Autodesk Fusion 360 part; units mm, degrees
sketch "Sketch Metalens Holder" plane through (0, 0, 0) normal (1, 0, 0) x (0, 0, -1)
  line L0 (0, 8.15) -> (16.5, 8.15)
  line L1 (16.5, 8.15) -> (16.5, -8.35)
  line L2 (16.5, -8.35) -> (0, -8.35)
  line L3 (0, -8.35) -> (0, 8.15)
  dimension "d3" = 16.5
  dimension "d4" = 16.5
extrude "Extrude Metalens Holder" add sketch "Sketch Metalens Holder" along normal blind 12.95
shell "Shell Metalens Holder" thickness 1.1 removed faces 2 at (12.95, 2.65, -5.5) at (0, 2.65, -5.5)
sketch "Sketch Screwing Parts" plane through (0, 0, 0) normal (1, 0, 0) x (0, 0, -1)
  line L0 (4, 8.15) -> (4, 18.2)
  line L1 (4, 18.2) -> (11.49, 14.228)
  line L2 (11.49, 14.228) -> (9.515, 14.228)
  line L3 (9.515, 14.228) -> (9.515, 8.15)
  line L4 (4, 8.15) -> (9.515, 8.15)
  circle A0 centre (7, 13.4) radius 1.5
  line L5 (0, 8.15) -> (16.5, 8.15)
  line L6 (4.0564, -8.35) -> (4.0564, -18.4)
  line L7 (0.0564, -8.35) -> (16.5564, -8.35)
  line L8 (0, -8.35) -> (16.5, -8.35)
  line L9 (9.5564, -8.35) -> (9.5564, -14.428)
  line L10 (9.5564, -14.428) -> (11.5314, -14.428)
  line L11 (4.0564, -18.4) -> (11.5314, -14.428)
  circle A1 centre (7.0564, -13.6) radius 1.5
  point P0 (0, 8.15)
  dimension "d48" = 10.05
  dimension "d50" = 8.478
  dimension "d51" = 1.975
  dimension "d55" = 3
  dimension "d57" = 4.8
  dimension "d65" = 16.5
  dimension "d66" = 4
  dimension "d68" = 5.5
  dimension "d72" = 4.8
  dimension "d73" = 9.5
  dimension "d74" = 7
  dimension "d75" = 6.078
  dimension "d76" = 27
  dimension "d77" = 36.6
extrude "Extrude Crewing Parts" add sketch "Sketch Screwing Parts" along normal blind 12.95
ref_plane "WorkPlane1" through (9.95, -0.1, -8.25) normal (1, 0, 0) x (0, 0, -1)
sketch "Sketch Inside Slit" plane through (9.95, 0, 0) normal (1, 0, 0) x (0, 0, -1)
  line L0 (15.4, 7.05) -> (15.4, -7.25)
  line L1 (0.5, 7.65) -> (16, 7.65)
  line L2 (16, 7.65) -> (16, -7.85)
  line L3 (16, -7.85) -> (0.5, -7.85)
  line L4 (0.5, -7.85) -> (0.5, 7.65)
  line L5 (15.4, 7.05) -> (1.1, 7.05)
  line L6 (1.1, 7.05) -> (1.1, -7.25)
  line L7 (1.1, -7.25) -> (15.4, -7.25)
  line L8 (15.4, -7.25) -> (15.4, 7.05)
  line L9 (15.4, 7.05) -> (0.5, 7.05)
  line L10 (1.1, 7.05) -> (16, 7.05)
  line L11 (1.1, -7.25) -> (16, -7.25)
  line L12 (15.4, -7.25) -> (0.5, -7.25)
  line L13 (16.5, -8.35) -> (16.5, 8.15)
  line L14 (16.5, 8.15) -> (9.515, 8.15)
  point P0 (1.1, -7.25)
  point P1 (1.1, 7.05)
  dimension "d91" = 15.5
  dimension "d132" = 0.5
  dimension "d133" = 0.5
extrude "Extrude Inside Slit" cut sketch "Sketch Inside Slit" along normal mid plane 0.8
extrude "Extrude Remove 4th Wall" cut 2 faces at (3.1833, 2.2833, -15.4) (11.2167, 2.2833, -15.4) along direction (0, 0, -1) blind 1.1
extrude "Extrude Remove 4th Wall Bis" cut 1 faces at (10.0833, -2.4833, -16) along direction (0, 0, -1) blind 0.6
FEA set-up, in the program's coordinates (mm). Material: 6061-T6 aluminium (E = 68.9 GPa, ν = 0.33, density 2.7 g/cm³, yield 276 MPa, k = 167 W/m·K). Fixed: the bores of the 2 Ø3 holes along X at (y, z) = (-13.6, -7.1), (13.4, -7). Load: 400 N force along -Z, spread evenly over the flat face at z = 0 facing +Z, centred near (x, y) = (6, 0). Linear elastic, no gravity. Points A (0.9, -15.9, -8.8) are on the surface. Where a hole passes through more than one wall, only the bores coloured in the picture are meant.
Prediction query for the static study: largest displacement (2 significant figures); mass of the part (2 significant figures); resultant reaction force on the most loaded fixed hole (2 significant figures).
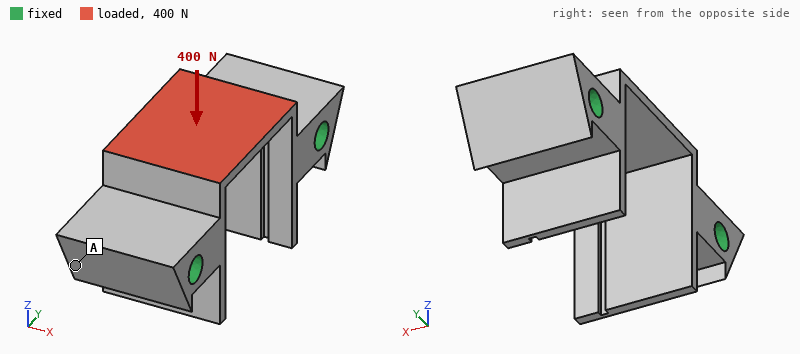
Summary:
52 µm
4.6 g
260 N
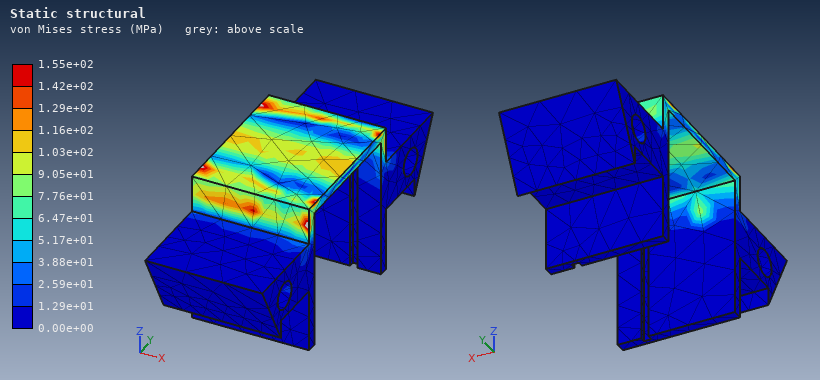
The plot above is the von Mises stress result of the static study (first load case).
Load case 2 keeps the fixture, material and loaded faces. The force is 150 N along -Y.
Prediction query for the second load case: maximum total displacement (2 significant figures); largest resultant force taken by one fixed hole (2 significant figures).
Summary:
10 µm
77 N
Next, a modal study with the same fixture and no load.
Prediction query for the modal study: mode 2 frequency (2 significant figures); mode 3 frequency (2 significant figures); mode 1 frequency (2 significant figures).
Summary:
16 kHz
22 kHz
16 kHz
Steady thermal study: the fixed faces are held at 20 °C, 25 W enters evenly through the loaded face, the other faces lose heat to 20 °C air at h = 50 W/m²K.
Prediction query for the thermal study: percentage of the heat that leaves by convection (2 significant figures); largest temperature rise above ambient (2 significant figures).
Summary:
3.2 %
45 K
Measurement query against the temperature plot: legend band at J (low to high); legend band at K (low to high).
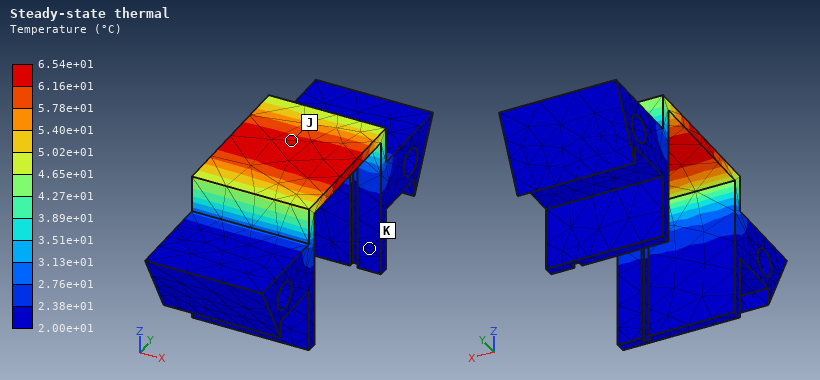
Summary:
6.16e+01 to 6.54e+01 °C
2.00e+01 to 2.38e+01 °C
